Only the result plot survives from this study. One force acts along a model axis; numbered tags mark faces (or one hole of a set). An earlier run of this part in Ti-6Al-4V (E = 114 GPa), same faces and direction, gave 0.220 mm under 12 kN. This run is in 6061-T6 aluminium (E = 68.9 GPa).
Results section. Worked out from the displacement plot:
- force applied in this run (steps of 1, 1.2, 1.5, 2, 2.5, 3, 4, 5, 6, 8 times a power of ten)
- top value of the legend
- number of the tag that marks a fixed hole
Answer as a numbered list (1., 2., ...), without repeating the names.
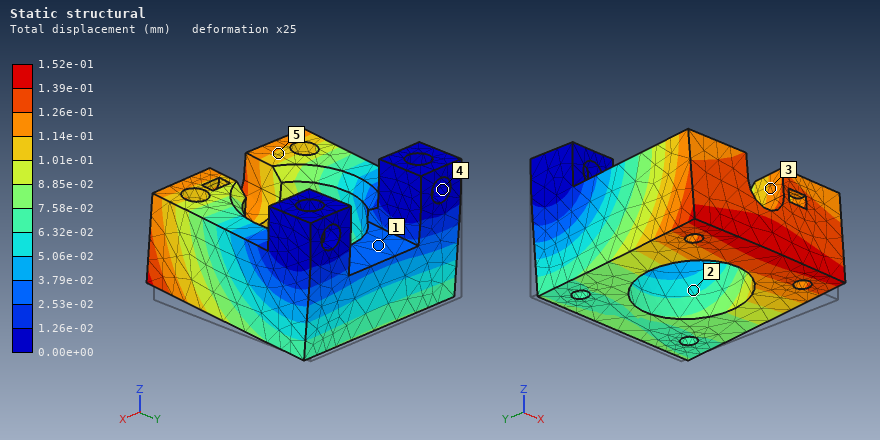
1. 5 kN
2. 1.52e-01 mm
3. 4
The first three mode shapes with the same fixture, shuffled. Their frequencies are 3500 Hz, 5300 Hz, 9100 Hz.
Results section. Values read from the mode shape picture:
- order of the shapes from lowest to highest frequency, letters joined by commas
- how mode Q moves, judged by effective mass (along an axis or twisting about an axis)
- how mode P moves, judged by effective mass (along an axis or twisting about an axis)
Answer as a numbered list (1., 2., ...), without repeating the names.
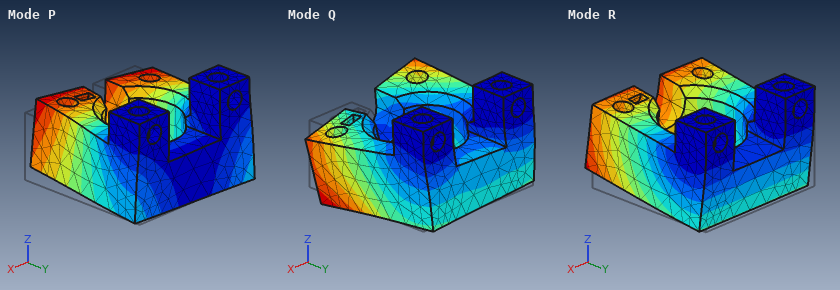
1. R, P, Q
2. along X
3. along X
